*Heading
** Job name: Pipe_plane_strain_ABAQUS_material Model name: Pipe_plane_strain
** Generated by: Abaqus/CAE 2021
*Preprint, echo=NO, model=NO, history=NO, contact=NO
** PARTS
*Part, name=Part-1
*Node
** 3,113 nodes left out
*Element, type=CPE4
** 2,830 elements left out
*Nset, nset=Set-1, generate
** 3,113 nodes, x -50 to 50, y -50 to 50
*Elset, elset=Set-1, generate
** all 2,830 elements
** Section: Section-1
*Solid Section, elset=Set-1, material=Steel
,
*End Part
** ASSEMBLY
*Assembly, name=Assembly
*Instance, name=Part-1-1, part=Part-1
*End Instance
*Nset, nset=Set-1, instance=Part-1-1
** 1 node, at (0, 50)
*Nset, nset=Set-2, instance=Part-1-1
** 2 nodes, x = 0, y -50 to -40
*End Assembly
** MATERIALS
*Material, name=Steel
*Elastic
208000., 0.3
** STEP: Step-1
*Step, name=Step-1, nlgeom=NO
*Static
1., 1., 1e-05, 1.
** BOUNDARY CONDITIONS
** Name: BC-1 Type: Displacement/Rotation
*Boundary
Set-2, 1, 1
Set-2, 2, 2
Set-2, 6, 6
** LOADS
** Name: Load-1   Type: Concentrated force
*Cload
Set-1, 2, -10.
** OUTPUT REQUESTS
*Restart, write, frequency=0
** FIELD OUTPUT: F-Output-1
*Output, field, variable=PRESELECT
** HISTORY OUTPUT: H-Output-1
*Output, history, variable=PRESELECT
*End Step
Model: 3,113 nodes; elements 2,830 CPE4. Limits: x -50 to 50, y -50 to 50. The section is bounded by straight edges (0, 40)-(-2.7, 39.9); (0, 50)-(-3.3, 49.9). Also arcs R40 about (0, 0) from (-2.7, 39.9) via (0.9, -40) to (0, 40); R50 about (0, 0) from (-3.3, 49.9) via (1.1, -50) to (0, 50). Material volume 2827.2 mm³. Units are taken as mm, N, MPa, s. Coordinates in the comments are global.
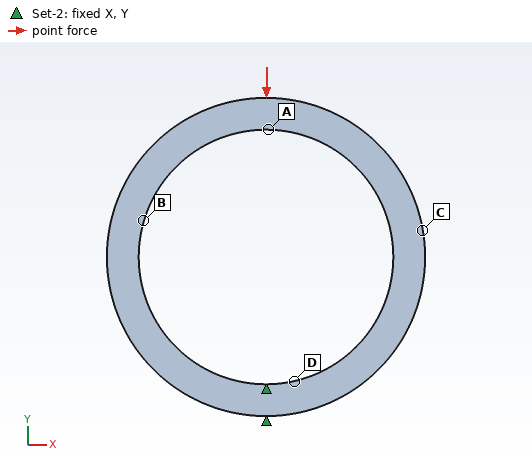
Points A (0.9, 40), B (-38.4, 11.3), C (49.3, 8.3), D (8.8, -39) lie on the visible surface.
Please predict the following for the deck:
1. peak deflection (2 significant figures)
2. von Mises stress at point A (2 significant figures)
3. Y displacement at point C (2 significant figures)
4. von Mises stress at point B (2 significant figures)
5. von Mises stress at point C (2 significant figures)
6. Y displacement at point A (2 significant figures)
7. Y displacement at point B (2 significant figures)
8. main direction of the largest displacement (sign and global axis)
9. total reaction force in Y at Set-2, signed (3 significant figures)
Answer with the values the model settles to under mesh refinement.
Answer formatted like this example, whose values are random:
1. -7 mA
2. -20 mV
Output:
1. 0.0077 mm
2. 7.9 MPa
3. -0.0037 mm
4. 4.7 MPa
5. 3.5 MPa
6. -0.0076 mm
7. -0.0042 mm
8. -Y
9. 10.0 N
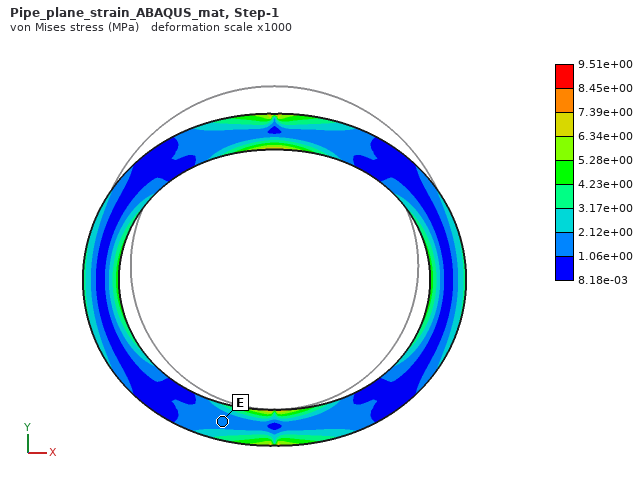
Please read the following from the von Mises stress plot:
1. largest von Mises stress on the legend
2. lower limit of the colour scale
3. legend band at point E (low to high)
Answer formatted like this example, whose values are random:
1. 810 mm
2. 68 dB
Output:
1. 9.51e+00 MPa
2. 8.18e-03 MPa
3. 1.06e+00 to 2.12e+00 MPa
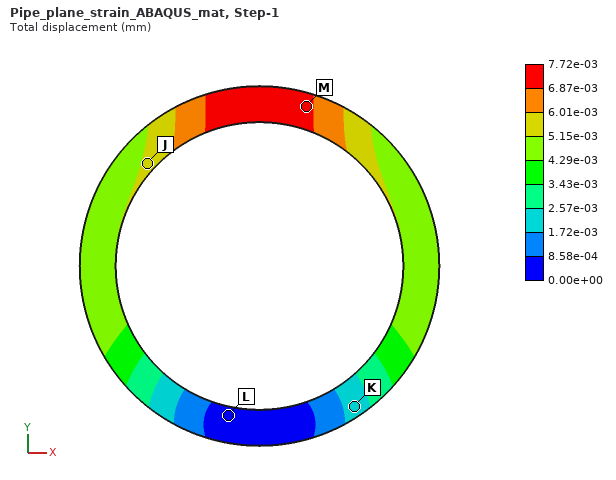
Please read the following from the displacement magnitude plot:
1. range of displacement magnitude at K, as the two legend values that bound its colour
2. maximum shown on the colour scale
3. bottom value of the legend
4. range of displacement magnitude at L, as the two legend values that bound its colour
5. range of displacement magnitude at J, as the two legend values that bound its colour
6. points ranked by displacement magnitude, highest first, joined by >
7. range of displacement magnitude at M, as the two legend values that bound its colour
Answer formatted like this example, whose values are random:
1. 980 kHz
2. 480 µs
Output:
1. 1.72e-03 to 2.57e-03 mm
2. 7.72e-03 mm
3. 0.00e+00 mm
4. 0.00e+00 to 8.58e-04 mm
5. 5.15e-03 to 6.01e-03 mm
6. M > J > K > L
7. 6.87e-03 to 7.72e-03 mm
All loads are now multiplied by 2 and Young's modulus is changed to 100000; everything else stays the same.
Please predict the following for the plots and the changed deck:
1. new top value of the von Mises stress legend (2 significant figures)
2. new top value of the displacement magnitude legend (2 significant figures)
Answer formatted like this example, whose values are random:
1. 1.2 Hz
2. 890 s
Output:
1. 19 MPa
2. 0.032 mm
